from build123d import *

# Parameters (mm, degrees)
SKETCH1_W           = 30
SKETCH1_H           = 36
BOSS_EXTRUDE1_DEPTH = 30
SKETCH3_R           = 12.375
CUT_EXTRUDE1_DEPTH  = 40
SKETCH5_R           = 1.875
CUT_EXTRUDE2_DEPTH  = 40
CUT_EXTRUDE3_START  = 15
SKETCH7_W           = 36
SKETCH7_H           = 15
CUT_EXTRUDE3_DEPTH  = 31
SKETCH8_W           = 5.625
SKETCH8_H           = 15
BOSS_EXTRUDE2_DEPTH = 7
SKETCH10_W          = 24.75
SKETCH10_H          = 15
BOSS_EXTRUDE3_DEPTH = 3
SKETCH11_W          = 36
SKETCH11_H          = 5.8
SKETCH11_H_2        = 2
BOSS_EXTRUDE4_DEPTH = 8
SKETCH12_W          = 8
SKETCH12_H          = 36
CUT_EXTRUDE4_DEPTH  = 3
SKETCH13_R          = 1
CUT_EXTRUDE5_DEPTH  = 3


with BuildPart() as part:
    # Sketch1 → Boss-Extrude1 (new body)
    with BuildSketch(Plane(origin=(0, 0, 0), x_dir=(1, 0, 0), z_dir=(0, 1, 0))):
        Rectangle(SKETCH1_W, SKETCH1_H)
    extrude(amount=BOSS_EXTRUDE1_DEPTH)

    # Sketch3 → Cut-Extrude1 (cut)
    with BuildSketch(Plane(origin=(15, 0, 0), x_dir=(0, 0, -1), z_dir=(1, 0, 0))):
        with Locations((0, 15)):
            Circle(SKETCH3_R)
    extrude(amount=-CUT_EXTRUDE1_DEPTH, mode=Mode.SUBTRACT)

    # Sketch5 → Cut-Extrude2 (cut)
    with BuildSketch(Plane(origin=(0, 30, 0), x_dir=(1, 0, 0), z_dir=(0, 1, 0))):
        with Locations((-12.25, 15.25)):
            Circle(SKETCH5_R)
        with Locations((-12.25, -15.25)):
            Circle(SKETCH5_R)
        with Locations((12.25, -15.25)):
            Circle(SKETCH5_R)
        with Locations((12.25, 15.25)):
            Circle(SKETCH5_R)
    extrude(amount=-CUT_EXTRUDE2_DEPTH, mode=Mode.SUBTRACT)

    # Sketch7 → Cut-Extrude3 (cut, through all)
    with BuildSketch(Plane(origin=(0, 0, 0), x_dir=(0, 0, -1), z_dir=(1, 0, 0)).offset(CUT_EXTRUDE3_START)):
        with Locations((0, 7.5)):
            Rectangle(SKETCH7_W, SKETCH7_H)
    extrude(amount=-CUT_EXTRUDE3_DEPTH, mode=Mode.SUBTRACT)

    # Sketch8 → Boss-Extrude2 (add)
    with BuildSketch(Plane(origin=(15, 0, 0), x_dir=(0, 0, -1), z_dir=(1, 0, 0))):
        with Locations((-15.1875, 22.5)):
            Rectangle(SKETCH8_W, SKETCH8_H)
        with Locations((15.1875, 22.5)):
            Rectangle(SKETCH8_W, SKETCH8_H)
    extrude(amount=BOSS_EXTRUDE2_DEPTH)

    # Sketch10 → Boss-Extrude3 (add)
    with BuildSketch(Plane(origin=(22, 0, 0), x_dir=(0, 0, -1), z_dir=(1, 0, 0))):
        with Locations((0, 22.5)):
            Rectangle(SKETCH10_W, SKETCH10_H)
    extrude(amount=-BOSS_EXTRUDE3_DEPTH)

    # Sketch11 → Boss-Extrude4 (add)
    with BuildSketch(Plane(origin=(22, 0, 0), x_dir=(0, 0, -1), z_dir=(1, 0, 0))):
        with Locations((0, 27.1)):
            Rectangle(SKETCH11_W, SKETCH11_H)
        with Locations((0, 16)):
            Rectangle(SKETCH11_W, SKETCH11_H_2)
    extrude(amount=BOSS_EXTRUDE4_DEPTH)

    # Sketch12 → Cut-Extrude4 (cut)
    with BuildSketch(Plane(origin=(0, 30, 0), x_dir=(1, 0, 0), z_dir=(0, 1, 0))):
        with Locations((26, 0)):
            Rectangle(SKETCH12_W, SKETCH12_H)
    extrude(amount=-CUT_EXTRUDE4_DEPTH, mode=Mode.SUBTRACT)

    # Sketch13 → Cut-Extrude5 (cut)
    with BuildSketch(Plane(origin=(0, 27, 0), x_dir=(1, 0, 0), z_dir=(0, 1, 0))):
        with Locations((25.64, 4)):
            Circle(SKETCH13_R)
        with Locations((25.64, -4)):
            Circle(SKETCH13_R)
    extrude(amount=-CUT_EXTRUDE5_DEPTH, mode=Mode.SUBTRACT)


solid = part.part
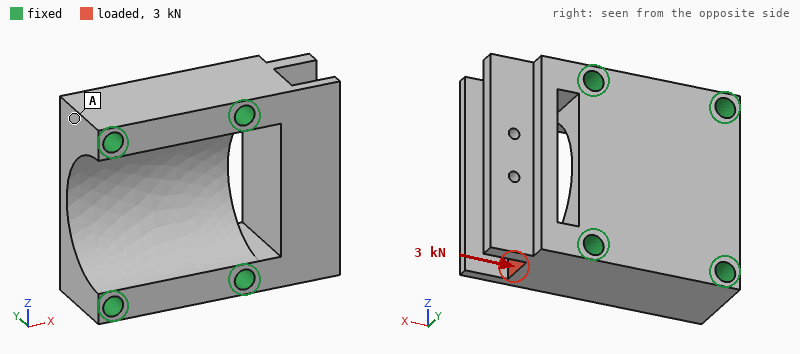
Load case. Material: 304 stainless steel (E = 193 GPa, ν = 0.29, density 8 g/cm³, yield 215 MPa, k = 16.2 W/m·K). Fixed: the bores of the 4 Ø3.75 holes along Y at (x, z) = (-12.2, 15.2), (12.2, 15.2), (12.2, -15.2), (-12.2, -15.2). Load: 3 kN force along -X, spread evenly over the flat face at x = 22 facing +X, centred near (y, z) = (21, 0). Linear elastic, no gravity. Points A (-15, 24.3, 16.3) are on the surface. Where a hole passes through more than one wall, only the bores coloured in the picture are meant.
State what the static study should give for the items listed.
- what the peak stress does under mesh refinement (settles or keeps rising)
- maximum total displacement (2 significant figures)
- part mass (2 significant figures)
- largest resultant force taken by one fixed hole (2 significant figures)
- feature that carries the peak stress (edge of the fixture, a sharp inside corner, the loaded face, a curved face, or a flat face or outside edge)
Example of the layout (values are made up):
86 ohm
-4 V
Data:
keeps rising
7.0 µm
96 g
1.6 kN
a sharp inside corner
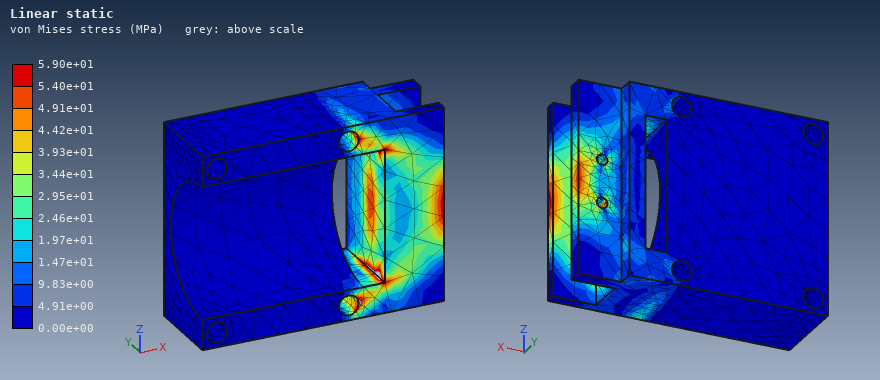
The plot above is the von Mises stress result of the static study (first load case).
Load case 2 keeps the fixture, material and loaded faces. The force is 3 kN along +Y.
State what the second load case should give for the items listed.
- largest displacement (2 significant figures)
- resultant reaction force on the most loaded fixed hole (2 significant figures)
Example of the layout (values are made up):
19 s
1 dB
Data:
13 µm
1.5 kN
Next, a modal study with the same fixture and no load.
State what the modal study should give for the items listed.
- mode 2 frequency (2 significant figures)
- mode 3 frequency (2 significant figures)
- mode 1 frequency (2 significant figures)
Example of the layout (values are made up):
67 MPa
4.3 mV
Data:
20 kHz
20 kHz
15 kHz
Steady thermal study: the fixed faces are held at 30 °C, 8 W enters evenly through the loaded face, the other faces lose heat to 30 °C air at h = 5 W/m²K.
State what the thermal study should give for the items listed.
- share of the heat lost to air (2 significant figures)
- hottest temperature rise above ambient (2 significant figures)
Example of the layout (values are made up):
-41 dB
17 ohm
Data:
4.0 %
43 K
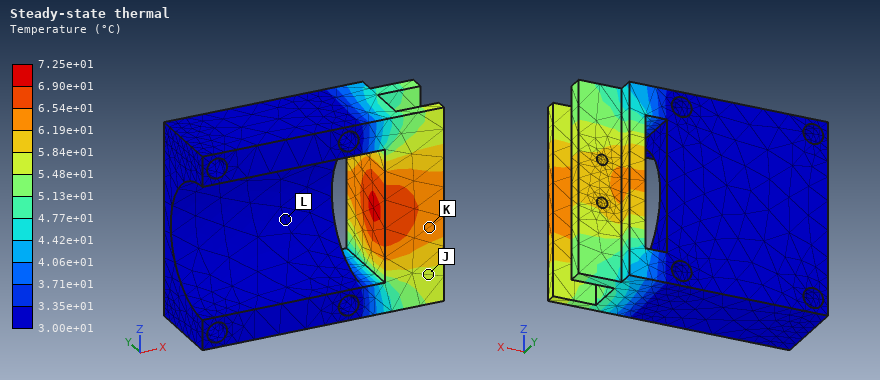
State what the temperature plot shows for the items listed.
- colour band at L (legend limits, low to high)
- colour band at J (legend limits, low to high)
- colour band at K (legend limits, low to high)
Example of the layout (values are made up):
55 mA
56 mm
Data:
3.00e+01 to 3.35e+01 °C
5.48e+01 to 5.84e+01 °C
6.19e+01 to 6.54e+01 °C
